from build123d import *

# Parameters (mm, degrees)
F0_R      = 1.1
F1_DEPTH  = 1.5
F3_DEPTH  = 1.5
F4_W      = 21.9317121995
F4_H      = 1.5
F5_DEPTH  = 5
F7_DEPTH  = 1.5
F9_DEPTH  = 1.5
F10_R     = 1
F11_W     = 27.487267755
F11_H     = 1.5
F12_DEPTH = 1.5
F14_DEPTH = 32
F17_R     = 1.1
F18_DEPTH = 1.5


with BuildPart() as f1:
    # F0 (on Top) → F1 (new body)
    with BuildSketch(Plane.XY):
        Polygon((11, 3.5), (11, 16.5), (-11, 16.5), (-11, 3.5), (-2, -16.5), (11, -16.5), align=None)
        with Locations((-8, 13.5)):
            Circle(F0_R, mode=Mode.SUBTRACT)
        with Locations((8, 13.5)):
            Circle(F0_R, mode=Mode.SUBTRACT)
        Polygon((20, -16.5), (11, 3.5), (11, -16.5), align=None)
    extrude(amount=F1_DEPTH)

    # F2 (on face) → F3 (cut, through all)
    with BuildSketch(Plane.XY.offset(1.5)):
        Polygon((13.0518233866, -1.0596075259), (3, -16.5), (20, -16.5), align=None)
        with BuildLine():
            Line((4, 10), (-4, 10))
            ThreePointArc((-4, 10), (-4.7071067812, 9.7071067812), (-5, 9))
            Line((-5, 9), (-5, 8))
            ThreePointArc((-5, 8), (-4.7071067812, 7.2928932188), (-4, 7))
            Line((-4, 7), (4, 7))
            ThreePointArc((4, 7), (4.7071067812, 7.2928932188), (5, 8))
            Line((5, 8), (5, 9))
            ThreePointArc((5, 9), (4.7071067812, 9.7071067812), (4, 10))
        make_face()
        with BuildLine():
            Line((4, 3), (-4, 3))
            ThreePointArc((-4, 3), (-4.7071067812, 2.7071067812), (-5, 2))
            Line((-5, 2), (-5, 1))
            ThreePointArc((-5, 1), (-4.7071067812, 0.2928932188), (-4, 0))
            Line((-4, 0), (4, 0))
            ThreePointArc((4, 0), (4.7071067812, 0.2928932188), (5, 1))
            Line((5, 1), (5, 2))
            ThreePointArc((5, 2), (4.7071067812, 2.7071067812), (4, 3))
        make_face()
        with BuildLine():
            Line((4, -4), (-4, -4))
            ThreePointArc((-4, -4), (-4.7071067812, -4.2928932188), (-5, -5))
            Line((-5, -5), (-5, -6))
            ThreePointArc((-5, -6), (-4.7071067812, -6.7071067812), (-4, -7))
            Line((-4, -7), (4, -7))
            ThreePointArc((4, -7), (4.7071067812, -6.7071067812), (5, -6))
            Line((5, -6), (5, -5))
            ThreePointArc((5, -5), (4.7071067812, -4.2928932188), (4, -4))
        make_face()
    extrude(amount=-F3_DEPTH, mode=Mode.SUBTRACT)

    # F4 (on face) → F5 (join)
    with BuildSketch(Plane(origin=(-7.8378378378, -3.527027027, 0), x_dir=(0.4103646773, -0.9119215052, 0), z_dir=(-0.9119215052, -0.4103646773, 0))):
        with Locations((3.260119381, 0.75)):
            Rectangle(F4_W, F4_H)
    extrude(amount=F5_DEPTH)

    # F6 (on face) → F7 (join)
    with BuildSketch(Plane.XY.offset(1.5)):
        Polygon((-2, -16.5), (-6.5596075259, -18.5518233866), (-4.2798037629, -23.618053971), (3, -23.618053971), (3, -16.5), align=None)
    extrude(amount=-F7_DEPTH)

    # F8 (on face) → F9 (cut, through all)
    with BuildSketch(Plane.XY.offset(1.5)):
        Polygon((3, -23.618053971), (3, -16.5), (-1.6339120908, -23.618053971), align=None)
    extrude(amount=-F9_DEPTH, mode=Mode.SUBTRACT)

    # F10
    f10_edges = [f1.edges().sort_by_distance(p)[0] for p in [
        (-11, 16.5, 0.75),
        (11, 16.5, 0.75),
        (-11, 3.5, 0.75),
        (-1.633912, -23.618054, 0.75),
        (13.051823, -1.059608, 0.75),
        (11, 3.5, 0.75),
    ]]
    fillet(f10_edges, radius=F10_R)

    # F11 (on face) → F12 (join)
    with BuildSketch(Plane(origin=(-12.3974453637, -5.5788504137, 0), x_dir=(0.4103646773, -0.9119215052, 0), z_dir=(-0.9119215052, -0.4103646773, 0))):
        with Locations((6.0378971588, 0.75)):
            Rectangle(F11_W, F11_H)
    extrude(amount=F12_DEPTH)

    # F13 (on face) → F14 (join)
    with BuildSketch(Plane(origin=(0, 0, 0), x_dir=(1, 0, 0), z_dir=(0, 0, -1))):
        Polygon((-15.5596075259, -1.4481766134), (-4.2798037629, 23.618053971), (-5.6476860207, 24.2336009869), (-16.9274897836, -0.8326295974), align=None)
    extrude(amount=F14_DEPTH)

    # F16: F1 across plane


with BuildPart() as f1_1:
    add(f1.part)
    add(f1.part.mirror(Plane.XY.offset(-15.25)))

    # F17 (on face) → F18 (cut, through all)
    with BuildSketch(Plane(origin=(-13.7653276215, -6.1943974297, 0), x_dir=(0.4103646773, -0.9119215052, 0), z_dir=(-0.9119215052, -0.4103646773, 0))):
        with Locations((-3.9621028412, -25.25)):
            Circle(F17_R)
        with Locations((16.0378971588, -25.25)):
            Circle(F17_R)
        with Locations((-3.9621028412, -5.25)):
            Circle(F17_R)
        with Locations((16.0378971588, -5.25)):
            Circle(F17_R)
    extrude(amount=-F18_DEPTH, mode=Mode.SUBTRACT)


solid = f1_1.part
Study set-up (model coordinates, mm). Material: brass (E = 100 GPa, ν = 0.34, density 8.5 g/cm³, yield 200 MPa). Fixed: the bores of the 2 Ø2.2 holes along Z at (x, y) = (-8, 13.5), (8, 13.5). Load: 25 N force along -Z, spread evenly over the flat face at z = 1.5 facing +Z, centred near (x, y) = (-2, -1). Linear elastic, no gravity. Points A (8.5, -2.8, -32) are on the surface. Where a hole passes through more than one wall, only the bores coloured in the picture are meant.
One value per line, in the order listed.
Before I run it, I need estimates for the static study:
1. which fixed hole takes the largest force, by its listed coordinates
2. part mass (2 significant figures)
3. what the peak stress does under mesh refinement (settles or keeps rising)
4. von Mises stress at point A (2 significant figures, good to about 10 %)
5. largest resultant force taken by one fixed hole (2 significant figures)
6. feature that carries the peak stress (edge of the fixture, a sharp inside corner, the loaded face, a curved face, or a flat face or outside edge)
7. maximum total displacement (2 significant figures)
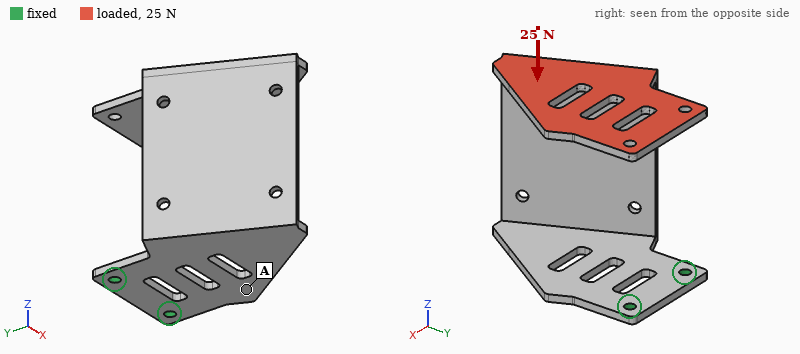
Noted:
(-8, 13.5)
28 g
keeps rising
9.0 MPa
15 N
edge of the fixture
0.63 mm
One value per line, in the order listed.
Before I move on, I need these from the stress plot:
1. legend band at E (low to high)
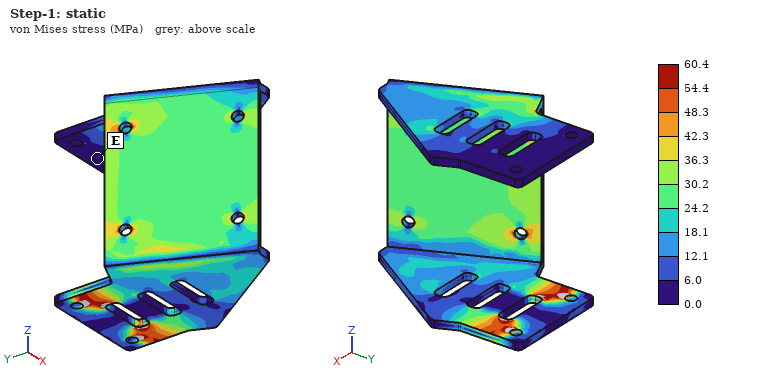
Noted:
0.0 to 6.0 MPa
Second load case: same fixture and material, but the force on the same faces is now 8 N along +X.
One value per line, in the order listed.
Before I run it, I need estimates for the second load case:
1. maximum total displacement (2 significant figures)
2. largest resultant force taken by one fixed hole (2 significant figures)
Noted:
0.47 mm
16 N
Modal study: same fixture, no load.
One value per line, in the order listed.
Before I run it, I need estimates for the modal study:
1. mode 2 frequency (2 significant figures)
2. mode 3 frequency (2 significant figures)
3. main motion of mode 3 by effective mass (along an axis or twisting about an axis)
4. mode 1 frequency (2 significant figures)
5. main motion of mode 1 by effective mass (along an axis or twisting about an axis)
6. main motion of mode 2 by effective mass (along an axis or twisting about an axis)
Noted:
230 Hz
530 Hz
along Z
160 Hz
along Y
along X
